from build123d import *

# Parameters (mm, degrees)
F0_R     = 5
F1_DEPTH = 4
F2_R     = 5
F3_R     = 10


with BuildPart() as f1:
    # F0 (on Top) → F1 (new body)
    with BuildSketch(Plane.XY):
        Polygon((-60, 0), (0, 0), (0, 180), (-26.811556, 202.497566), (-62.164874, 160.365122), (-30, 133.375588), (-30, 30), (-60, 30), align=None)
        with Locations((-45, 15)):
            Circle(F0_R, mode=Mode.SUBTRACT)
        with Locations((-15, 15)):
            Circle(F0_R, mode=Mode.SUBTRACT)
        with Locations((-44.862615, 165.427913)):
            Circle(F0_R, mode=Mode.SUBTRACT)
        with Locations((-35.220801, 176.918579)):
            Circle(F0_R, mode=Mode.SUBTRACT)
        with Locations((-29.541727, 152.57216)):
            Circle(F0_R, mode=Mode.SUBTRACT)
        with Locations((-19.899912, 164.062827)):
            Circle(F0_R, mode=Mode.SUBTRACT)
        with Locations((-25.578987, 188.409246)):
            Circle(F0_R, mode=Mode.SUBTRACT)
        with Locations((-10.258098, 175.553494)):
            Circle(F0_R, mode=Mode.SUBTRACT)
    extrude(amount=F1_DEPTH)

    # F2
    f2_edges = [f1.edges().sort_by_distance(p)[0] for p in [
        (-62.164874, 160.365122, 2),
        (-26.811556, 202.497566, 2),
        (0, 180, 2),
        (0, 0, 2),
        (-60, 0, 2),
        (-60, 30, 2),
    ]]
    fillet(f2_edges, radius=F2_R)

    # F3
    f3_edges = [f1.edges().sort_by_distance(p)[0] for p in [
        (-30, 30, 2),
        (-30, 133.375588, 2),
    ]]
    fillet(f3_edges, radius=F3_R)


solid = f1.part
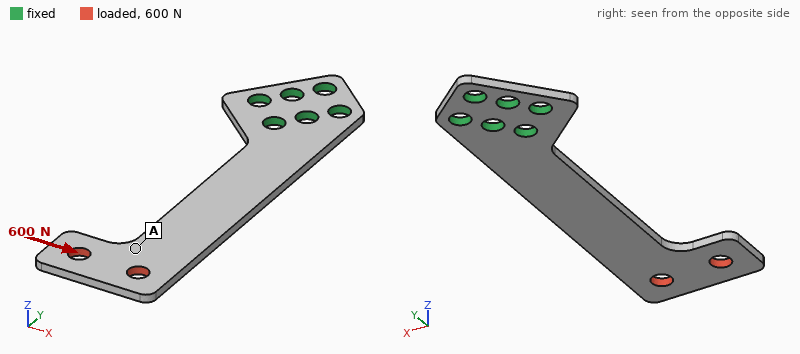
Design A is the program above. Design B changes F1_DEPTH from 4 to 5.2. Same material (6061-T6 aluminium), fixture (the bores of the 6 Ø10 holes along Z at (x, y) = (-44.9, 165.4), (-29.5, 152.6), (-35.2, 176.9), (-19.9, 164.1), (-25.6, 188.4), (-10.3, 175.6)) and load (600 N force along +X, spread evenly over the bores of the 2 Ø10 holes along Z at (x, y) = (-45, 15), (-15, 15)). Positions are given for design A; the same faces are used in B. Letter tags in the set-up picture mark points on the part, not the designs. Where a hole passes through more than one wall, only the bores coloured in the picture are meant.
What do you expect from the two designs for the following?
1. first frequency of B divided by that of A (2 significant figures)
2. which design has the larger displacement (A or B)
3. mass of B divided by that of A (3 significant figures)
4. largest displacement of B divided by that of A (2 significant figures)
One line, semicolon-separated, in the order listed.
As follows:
1.3; A; 1.30; 0.77
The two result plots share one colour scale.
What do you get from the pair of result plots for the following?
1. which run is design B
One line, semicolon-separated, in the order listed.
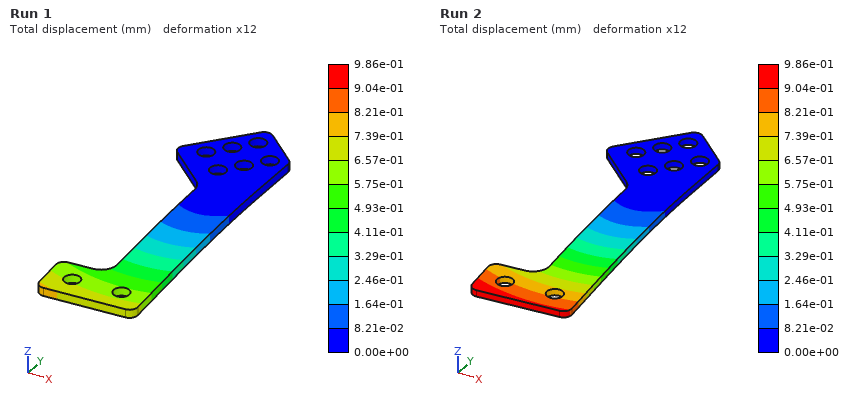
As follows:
Run 1
